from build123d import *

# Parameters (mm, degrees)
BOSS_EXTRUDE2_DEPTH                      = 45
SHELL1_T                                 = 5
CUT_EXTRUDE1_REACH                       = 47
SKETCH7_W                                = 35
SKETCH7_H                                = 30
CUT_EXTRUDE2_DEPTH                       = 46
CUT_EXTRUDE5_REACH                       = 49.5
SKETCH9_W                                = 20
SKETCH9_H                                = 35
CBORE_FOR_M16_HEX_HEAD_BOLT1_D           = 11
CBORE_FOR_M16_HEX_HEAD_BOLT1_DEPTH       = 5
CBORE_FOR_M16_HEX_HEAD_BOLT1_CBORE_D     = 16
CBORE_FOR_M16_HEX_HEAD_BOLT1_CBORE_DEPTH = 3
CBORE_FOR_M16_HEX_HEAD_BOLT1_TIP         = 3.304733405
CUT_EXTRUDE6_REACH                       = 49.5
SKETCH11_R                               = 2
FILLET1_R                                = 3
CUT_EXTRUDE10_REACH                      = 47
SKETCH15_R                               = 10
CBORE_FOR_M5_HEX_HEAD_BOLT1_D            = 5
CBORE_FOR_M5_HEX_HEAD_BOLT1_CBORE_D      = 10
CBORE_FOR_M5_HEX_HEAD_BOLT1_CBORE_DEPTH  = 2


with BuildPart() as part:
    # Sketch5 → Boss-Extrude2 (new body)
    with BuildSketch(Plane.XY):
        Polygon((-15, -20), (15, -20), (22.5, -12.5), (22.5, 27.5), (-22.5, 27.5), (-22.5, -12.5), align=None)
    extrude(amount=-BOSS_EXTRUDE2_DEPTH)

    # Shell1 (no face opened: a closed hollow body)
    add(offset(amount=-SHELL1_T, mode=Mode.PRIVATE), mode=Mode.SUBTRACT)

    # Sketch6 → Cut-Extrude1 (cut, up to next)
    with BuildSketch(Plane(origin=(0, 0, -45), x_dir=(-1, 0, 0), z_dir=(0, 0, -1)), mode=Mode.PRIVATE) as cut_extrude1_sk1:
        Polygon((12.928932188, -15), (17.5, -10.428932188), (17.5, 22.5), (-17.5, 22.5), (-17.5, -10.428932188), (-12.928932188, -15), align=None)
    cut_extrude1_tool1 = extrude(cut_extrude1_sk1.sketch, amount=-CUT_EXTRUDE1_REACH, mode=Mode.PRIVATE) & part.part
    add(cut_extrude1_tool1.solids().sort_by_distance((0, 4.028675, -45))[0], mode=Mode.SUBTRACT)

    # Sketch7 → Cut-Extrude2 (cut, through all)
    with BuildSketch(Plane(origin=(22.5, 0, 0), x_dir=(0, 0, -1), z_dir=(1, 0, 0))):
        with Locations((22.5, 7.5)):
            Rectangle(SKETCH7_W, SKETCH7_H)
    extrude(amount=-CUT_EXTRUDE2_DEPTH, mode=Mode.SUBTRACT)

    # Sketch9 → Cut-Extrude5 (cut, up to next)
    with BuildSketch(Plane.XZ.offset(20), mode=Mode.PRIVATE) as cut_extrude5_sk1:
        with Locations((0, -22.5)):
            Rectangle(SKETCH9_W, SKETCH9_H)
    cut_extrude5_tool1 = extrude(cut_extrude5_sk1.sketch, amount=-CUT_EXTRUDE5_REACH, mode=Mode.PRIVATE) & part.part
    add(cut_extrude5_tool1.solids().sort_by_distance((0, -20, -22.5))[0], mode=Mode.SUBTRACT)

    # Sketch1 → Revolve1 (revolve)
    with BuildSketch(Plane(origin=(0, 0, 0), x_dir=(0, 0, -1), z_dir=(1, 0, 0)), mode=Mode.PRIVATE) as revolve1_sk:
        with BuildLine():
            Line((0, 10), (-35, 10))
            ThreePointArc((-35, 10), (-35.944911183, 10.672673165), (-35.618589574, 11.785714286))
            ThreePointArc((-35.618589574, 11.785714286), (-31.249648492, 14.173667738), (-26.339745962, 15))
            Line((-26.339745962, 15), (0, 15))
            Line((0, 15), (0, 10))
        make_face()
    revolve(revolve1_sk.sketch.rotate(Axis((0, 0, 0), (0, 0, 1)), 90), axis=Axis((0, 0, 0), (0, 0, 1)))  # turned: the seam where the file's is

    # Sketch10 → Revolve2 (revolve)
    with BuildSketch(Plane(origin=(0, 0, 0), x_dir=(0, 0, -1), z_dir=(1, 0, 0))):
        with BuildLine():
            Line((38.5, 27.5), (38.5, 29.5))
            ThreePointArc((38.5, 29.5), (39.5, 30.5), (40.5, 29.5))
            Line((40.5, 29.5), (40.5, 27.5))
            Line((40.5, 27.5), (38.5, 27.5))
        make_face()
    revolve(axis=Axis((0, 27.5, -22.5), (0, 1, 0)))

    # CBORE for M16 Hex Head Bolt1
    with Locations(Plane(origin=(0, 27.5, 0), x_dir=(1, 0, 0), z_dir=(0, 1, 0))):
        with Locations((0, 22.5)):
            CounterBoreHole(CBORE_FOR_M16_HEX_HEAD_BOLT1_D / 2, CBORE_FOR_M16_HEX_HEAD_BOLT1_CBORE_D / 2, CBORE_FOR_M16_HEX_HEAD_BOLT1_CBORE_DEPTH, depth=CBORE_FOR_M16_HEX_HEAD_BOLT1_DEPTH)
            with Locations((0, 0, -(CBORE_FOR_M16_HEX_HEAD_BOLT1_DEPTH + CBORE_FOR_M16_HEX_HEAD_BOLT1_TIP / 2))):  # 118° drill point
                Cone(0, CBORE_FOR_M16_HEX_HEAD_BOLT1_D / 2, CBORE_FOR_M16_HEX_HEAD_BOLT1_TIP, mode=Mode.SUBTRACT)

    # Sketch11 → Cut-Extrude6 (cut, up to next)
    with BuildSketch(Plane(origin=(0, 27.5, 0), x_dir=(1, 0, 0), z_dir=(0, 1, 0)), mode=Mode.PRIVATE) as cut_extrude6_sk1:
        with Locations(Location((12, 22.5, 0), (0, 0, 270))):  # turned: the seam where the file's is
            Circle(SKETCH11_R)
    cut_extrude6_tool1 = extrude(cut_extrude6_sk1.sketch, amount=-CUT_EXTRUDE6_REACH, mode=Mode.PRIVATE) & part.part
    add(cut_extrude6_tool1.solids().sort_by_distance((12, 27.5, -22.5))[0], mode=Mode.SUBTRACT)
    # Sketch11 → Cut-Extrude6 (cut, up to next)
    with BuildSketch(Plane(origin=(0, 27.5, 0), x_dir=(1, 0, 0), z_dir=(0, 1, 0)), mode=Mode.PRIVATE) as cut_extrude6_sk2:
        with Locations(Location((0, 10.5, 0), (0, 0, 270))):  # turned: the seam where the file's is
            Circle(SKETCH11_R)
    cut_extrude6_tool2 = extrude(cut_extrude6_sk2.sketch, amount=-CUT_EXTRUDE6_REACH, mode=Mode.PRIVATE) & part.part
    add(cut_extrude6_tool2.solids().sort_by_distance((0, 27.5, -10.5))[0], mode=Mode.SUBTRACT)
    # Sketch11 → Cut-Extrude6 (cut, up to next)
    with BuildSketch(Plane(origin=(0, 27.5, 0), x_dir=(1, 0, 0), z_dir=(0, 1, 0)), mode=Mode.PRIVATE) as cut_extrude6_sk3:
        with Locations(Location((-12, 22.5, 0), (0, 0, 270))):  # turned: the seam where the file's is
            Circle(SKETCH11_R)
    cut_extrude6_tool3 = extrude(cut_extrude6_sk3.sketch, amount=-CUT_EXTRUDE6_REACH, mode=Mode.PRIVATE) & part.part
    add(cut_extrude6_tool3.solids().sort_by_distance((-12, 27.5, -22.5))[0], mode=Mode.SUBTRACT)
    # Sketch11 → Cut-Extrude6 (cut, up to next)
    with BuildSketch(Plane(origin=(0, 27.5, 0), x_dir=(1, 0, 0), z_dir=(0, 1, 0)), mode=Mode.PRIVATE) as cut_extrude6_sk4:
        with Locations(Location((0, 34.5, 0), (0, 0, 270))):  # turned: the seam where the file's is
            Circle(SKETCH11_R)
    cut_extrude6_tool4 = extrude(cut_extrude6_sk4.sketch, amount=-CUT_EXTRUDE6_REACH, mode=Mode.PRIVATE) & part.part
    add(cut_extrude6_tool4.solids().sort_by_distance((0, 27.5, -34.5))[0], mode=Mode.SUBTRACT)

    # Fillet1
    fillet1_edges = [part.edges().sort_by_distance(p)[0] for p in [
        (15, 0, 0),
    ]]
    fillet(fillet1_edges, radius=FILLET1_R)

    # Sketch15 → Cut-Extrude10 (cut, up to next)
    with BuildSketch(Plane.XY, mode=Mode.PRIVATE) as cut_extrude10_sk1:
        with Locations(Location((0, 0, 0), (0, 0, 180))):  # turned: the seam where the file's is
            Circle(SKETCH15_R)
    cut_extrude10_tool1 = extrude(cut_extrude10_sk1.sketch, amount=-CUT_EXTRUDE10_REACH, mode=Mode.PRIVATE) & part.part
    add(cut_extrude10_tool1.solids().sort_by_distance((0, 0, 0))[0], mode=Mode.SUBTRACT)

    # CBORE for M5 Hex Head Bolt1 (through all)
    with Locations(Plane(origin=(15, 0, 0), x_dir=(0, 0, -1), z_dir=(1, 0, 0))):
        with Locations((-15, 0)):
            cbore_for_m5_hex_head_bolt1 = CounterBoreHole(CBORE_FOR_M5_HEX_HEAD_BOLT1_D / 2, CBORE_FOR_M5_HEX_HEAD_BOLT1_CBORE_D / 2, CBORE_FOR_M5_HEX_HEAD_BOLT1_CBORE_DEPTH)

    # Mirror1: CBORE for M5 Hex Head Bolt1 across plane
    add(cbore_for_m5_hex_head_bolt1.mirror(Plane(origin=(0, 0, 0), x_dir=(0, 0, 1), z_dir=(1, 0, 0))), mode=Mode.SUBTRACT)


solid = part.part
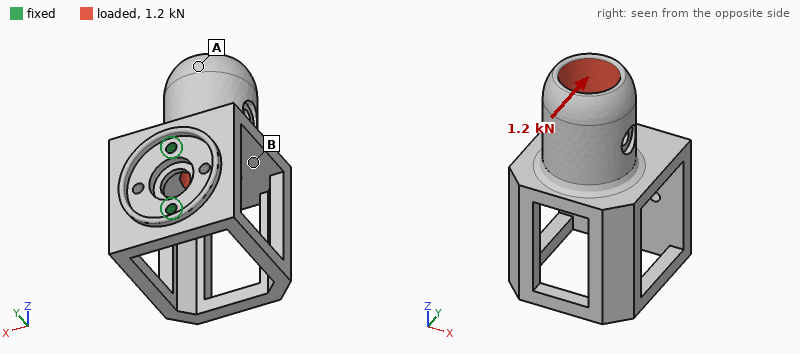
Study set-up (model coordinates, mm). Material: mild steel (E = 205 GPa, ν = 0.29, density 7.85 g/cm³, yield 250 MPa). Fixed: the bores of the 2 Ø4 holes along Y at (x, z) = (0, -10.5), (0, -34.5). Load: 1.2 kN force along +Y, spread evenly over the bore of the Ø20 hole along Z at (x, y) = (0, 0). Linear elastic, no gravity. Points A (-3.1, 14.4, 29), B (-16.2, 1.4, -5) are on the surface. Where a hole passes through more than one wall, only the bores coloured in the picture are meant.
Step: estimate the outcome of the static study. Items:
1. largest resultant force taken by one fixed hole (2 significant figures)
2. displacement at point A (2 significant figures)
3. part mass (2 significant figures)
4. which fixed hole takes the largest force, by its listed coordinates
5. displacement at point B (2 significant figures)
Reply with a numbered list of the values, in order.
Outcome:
1. 1.9 kN
2. 62 µm
3. 310 g
4. (0, -10.5)
5. 35 µm
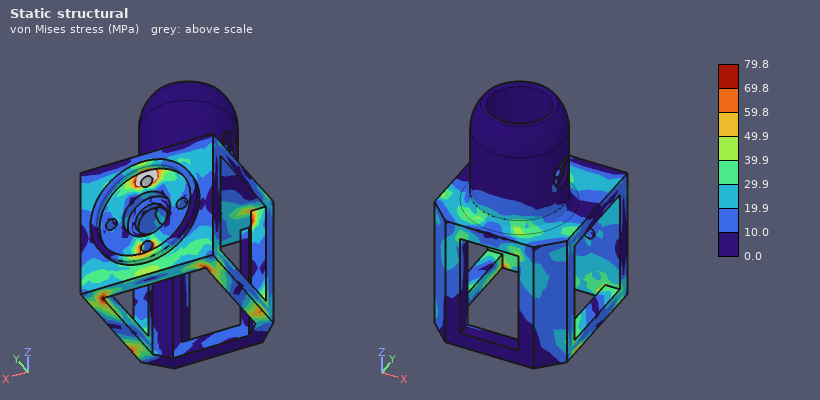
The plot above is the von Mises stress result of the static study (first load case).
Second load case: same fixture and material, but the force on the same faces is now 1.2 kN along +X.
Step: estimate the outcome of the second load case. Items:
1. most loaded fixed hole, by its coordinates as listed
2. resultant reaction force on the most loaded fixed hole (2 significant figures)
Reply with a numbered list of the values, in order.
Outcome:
1. (0, -10.5)
2. 2.1 kN
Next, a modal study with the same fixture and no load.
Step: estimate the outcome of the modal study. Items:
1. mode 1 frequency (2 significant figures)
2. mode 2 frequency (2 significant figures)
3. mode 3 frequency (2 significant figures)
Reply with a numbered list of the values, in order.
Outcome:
1. 1300 Hz
2. 1300 Hz
3. 2300 Hz
